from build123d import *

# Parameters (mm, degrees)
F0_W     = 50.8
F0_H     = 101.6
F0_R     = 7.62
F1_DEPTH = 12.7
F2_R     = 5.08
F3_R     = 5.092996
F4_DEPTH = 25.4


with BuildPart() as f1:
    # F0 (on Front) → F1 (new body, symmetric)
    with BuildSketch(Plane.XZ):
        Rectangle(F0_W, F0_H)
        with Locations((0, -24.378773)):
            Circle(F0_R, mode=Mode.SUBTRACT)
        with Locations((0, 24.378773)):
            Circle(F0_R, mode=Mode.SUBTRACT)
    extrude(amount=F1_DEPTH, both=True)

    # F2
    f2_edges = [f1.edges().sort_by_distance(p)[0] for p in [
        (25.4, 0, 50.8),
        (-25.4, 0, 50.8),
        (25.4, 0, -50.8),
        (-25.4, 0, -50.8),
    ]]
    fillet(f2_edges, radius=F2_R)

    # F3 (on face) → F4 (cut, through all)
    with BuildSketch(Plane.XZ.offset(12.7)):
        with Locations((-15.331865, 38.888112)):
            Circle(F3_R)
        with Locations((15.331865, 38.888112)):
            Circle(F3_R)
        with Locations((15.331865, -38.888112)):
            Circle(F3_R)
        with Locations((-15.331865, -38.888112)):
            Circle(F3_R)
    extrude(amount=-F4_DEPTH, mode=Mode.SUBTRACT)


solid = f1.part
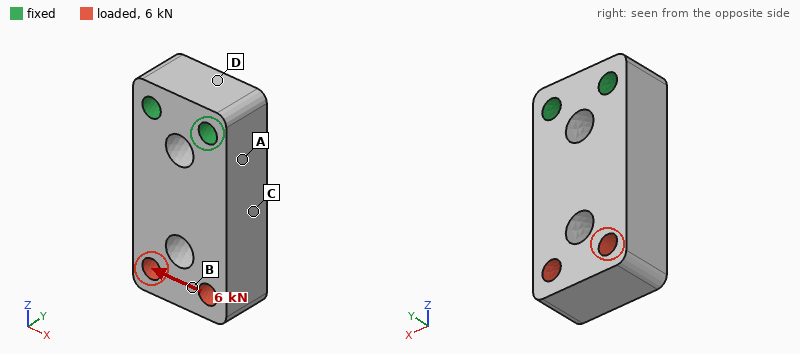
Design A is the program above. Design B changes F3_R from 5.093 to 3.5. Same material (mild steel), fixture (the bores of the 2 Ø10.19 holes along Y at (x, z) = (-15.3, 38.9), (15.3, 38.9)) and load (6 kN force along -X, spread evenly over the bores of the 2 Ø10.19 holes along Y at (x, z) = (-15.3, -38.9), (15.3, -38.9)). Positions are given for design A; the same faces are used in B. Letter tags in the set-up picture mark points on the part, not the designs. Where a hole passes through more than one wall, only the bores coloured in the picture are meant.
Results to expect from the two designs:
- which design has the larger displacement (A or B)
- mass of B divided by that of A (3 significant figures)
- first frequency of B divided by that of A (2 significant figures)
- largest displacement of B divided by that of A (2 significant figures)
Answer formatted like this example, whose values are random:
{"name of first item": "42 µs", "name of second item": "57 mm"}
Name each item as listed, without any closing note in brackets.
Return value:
{"which design has the larger displacement": "B", "mass of B divided by that of A": "1.04", "first frequency of B divided by that of A": "0.92", "largest displacement of B divided by that of A": "1.1"}
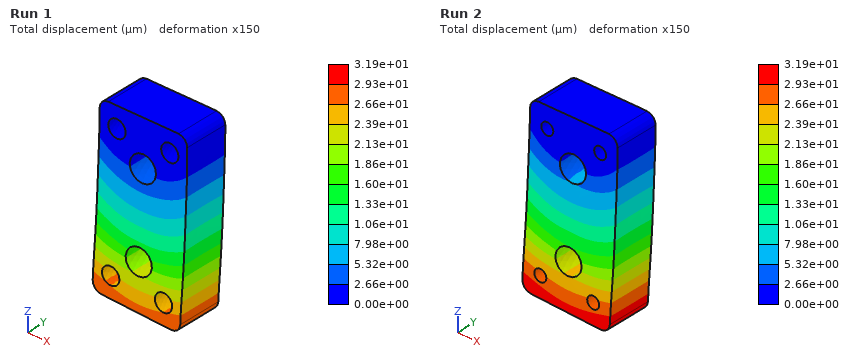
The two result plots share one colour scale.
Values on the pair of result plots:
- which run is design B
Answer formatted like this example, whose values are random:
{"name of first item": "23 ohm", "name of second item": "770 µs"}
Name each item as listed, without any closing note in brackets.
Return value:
{"which run is design B": "Run 2"}
